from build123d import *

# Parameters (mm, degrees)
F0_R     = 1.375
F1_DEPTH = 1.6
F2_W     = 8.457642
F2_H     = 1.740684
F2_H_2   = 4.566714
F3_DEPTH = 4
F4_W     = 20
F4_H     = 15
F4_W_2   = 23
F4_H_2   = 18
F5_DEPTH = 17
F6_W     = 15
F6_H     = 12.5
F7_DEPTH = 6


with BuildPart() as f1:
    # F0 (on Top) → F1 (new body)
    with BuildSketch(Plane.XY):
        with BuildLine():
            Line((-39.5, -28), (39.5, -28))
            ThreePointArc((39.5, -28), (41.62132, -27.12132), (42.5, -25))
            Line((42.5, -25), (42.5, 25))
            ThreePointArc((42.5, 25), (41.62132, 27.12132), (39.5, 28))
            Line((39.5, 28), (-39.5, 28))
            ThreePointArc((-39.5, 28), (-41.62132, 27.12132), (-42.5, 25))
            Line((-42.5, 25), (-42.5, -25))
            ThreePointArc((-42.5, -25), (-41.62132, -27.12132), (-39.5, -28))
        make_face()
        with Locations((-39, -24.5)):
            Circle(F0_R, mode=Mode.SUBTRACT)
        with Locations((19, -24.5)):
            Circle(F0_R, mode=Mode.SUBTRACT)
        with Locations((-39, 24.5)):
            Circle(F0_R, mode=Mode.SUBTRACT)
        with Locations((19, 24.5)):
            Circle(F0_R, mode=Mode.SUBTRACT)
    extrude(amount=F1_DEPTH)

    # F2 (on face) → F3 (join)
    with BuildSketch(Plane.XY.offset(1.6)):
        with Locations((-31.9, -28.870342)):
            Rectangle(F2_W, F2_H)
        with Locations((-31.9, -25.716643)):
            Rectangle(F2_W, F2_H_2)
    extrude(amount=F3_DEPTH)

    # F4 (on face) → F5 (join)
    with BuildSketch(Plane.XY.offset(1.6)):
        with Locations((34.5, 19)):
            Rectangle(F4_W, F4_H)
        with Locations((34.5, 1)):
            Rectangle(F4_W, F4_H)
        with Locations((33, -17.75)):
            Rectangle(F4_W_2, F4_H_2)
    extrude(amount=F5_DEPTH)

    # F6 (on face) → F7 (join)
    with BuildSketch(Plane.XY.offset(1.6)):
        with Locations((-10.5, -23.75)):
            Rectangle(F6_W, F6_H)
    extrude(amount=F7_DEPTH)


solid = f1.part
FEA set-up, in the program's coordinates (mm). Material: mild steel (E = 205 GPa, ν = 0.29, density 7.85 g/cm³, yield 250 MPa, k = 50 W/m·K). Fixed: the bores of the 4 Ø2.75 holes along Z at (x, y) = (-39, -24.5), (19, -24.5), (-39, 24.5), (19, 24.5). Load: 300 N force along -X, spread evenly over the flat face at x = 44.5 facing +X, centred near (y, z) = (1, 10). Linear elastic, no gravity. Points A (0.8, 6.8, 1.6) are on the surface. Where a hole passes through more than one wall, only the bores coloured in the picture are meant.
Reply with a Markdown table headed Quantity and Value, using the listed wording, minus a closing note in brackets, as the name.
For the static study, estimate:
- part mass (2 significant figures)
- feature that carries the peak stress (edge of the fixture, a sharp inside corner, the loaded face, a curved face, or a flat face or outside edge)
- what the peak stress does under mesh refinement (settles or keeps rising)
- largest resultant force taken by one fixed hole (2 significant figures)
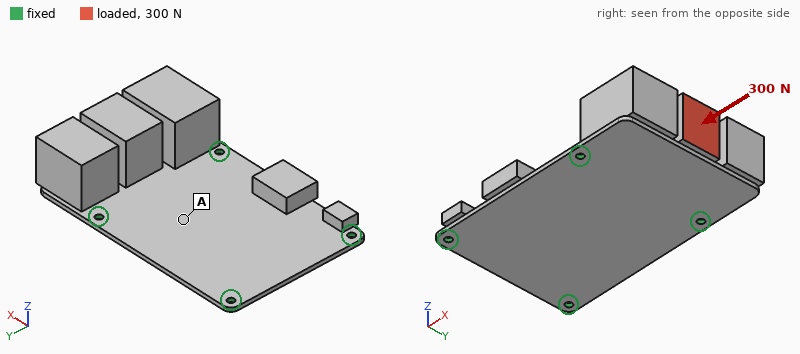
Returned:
| Quantity | Value |
|---|---|
| part mass | 210 g |
| feature that carries the peak stress | edge of the fixture |
| what the peak stress does under mesh refinement | keeps rising |
| largest resultant force taken by one fixed hole | 130 N |
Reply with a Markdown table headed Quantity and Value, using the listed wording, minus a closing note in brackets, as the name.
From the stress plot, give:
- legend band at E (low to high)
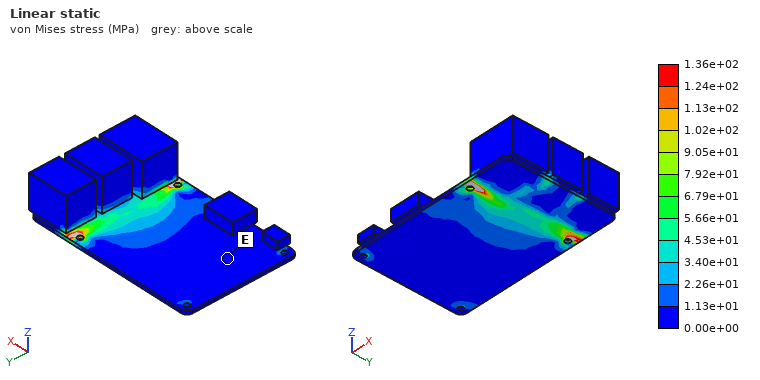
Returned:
| Quantity | Value |
|---|---|
| legend band at E | 0.00e+00 to 1.13e+01 MPa |
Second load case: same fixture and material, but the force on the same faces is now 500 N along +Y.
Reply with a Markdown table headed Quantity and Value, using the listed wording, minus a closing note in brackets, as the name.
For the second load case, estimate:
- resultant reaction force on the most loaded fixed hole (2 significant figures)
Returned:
| Quantity | Value |
|---|---|
| resultant reaction force on the most loaded fixed hole | 380 N |
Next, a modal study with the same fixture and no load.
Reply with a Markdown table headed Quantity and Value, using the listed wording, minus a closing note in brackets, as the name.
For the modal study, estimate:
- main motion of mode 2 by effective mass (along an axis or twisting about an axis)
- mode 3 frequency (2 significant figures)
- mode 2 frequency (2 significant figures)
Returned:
| Quantity | Value |
|---|---|
| main motion of mode 2 by effective mass | along Z |
| mode 3 frequency | 2000 Hz |
| mode 2 frequency | 1600 Hz |
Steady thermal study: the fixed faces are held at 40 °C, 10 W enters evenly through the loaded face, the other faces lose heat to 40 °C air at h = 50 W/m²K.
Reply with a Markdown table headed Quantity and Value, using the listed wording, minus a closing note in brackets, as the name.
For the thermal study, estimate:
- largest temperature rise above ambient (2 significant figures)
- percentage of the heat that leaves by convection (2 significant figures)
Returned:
| Quantity | Value |
|---|---|
| largest temperature rise above ambient | 35 K |
| percentage of the heat that leaves by convection | 62 % |
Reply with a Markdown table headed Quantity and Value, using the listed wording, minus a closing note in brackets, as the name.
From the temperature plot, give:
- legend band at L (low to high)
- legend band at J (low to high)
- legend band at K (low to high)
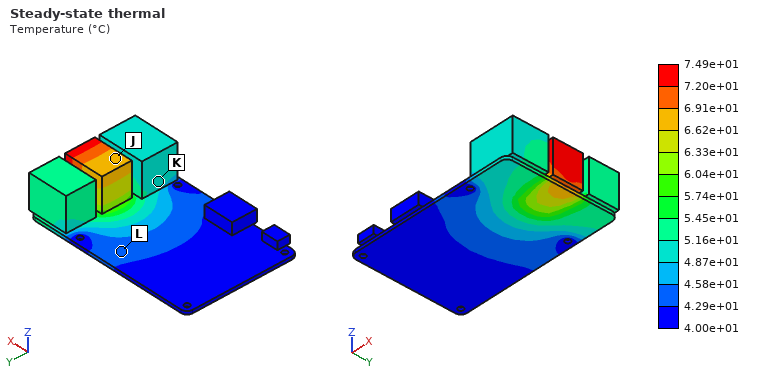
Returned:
| Quantity | Value |
|---|---|
| legend band at L | 4.29e+01 to 4.58e+01 °C |
| legend band at J | 6.62e+01 to 6.91e+01 °C |
| legend band at K | 4.87e+01 to 5.16e+01 °C |
